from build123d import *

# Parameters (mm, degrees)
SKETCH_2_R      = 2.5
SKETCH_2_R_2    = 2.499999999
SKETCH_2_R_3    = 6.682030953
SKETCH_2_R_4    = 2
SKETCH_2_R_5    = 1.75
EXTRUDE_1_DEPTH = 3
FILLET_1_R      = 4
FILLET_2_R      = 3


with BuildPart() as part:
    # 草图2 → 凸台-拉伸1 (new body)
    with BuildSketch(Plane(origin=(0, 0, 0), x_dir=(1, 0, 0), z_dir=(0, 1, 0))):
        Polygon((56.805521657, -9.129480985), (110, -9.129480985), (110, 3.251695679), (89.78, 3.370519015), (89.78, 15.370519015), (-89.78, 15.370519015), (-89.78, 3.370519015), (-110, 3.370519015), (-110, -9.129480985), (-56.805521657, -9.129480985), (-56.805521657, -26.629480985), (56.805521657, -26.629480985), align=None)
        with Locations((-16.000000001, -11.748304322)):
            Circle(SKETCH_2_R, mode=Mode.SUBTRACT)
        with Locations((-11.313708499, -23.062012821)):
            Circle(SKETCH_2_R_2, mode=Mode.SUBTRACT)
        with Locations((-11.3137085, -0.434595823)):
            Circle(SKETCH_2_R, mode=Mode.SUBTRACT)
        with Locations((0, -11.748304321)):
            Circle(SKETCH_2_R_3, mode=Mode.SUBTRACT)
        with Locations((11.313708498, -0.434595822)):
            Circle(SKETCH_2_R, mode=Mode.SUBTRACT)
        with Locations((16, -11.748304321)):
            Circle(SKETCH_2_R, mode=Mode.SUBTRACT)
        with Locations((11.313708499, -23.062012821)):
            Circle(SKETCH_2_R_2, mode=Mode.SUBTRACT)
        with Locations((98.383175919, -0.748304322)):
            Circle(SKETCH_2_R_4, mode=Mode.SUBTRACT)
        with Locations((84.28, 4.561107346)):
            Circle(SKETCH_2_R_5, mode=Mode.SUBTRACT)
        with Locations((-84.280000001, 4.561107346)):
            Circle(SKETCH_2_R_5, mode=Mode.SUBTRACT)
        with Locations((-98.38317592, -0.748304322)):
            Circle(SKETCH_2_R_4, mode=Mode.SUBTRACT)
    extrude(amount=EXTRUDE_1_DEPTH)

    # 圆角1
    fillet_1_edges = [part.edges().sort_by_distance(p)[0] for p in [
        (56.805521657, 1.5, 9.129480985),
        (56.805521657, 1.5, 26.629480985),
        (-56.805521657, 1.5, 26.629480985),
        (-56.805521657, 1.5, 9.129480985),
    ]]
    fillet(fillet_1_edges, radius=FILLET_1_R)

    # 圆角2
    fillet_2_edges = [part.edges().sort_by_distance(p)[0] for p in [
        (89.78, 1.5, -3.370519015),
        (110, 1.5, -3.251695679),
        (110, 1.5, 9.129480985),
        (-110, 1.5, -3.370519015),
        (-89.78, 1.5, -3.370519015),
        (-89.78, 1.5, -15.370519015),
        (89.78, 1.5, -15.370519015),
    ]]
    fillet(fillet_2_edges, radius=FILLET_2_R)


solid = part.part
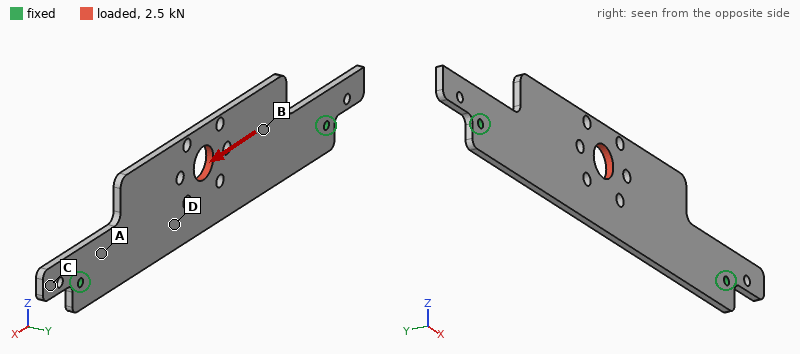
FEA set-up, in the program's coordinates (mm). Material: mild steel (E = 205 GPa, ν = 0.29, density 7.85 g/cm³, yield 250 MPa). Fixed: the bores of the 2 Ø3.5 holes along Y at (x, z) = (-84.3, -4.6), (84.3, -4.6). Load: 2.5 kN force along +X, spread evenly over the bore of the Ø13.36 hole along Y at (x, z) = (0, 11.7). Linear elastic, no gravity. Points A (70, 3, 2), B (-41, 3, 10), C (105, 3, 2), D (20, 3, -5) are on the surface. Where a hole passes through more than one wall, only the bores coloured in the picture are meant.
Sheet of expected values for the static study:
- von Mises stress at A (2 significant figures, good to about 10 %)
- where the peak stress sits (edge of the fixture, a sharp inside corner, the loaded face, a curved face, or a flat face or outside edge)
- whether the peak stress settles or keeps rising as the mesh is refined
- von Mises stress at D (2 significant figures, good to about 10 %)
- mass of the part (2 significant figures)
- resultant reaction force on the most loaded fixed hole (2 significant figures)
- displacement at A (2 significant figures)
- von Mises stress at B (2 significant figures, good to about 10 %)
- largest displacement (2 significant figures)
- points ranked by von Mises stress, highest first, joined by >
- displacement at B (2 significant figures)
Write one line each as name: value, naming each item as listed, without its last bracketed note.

von Mises stress at A: 23 MPa
where the peak stress sits: edge of the fixture
whether the peak stress settles or keeps rising as the mesh is refined: keeps rising
von Mises stress at D: 8.6 MPa
mass of the part: 160 g
resultant reaction force on the most loaded fixed hole: 1.3 kN
displacement at A: 2.1 µm
von Mises stress at B: 14 MPa
largest displacement: 8.6 µm
points ranked by von Mises stress, highest first, joined by >: A > B > D > C
displacement at B: 4.9 µm
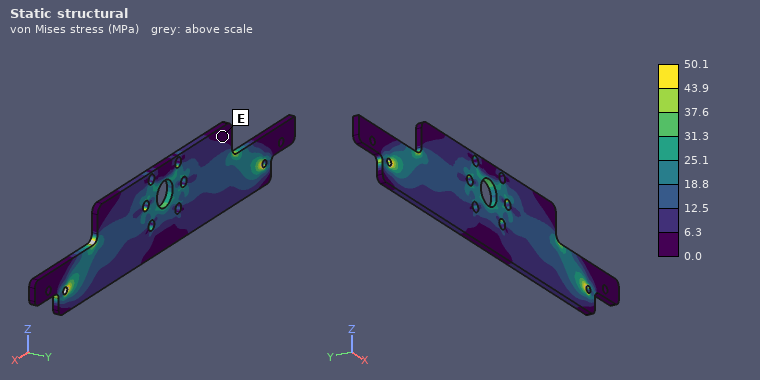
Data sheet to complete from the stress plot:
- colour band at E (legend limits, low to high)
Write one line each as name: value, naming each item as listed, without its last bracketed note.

colour band at E: 0.0 to 6.3 MPa
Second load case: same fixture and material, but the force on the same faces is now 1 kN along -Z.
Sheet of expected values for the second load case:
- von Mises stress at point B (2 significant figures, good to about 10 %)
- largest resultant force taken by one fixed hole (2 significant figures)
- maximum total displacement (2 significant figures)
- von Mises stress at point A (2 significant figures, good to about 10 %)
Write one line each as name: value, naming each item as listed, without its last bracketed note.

von Mises stress at point B: 18 MPa
largest resultant force taken by one fixed hole: 760 N
maximum total displacement: 32 µm
von Mises stress at point A: 20 MPa
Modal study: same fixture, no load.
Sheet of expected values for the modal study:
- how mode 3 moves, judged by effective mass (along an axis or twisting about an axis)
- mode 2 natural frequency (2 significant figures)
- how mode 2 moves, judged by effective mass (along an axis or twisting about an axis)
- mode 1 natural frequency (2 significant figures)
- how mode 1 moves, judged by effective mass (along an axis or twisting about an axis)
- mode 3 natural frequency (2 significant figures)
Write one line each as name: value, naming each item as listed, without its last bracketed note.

how mode 3 moves, judged by effective mass: twisting about Z
mode 2 natural frequency: 1100 Hz
how mode 2 moves, judged by effective mass: twisting about X
mode 1 natural frequency: 450 Hz
how mode 1 moves, judged by effective mass: along Y
mode 3 natural frequency: 1300 Hz
